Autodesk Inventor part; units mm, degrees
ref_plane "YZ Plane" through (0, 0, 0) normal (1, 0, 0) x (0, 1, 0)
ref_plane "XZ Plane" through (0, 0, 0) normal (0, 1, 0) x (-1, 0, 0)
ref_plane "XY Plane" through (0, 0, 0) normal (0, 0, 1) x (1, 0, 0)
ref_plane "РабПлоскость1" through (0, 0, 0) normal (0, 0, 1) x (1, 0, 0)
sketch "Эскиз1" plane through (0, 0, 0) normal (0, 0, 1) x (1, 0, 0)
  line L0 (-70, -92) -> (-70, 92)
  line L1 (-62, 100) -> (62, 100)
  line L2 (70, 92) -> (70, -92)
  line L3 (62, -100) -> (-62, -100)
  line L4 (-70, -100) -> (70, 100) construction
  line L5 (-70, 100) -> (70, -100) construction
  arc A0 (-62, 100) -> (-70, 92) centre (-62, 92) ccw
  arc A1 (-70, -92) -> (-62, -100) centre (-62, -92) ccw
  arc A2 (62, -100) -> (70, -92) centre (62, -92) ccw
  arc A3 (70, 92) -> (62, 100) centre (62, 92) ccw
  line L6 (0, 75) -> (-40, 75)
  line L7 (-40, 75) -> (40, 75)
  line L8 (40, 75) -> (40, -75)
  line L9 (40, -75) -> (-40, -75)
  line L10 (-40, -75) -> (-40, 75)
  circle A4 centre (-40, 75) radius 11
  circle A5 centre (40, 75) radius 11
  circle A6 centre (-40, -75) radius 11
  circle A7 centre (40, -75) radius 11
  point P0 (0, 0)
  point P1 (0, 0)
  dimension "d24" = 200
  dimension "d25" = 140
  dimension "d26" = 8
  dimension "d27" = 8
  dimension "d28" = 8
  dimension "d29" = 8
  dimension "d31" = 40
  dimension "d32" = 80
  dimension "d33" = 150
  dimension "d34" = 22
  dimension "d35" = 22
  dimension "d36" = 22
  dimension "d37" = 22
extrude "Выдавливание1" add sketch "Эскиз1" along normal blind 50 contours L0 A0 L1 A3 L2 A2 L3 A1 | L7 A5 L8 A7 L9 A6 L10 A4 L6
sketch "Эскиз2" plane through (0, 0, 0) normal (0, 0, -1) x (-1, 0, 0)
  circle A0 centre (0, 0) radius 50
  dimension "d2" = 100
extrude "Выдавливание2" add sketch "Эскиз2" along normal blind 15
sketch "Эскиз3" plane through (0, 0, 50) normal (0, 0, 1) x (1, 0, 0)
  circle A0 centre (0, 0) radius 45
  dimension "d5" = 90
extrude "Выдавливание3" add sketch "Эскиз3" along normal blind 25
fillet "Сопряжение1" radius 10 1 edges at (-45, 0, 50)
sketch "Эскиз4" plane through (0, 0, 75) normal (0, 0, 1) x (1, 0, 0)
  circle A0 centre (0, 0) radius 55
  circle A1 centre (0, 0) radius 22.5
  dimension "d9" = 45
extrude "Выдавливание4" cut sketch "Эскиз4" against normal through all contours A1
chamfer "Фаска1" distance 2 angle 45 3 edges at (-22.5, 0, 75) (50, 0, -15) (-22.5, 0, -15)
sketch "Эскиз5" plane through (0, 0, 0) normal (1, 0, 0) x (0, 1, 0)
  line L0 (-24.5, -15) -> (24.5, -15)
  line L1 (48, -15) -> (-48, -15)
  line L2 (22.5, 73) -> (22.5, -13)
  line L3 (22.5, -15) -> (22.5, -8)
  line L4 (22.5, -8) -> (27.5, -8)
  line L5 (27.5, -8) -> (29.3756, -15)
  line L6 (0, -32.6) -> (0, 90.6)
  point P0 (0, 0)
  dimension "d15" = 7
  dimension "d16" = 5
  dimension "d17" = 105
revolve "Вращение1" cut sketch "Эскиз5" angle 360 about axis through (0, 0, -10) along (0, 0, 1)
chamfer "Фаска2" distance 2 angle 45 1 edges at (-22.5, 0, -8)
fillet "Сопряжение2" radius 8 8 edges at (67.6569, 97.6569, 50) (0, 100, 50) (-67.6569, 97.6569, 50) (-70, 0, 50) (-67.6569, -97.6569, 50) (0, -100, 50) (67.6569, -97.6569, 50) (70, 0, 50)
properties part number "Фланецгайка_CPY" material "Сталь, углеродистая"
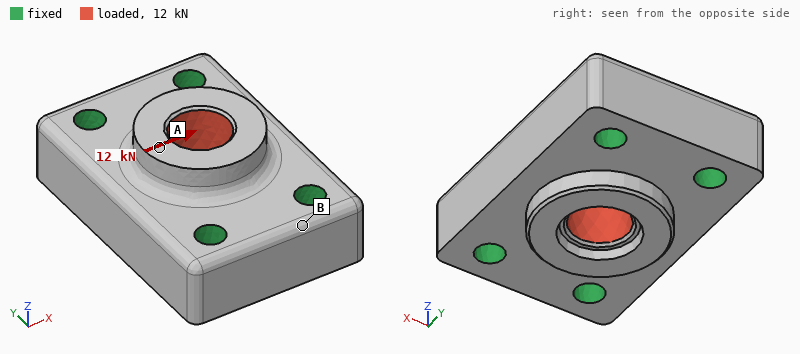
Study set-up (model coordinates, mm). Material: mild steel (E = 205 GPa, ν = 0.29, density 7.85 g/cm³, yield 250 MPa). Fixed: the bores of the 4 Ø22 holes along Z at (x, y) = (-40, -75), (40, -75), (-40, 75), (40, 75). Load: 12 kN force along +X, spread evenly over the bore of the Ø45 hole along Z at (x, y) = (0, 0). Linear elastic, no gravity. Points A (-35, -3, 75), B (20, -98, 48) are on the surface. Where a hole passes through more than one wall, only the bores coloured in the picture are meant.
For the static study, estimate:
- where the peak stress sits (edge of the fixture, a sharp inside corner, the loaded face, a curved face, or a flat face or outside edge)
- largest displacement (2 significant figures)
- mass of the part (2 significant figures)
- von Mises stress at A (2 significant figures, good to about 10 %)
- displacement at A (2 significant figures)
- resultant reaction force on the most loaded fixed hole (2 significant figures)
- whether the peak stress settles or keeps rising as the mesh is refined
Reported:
edge of the fixture
1.1 µm
11 kg
1.2 MPa
1.1 µm
3.5 kN
keeps rising
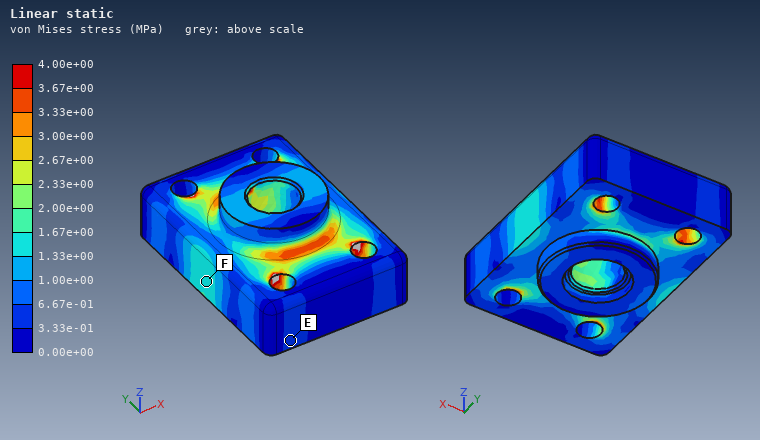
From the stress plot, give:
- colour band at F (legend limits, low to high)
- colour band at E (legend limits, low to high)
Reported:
1.33e+00 to 1.67e+00 MPa
3.33e-01 to 6.67e-01 MPa
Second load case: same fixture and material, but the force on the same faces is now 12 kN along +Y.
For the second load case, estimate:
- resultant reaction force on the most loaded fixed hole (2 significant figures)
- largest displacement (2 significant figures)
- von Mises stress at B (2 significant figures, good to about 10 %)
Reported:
3.1 kN
0.65 µm
0.29 MPa
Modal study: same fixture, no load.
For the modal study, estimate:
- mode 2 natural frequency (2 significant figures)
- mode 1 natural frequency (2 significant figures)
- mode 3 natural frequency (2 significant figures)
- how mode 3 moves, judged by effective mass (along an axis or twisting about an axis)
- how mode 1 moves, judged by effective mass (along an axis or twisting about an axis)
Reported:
8100 Hz
7600 Hz
9200 Hz
along X
along Z
